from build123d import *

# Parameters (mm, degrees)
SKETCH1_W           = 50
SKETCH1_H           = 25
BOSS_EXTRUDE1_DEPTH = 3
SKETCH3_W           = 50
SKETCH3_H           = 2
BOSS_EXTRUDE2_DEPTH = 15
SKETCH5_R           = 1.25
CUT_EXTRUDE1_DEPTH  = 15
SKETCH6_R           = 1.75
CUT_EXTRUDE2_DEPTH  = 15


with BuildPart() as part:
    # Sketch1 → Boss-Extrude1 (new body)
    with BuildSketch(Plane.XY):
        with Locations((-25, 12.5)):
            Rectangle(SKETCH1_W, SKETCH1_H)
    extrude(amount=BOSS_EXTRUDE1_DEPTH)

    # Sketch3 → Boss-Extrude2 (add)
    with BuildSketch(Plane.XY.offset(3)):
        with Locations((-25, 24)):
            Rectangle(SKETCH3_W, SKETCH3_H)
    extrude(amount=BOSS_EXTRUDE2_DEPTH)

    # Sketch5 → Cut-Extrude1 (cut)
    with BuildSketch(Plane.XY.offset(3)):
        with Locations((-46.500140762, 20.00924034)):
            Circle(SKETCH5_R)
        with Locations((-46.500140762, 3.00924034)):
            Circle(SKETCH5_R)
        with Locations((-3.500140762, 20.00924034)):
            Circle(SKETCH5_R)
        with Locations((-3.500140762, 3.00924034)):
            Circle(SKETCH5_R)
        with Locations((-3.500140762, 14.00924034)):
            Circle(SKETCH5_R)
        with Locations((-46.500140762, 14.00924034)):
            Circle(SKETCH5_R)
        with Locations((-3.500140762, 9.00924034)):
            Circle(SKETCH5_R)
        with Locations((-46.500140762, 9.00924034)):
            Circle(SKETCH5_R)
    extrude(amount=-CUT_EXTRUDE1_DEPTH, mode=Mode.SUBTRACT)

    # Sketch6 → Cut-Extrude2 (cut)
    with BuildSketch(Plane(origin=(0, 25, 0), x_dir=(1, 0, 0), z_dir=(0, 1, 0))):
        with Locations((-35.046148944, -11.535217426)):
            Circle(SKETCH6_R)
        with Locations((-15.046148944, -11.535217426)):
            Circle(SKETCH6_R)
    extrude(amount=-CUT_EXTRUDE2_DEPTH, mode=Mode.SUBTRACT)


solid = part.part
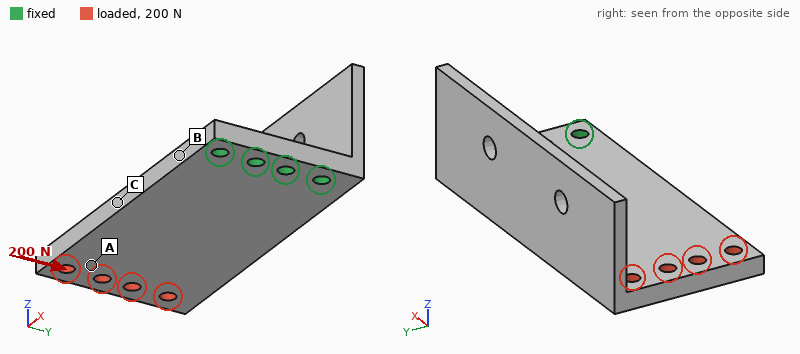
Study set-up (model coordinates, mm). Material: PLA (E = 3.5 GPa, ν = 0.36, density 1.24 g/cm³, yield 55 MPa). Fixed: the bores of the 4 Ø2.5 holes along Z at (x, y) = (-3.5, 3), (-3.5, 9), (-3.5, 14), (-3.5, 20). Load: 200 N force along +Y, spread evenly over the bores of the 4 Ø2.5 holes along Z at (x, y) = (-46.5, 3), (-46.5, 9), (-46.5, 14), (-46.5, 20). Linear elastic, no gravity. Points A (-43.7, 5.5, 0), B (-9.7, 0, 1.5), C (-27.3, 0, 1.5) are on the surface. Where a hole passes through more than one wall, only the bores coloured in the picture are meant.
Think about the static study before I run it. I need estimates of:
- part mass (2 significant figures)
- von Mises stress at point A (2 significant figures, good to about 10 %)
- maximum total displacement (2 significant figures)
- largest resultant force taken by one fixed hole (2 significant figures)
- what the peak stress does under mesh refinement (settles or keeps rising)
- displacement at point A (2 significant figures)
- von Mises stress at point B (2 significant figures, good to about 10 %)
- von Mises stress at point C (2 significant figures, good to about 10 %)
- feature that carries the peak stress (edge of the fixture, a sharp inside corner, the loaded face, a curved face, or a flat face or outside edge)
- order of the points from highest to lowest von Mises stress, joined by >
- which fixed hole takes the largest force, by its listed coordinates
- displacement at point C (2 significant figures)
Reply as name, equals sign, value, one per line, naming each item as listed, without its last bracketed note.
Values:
part mass = 6.3 g
von Mises stress at point A = 4.5 MPa
maximum total displacement = 0.60 mm
largest resultant force taken by one fixed hole = 470 N
what the peak stress does under mesh refinement = keeps rising
displacement at point A = 0.48 mm
von Mises stress at point B = 22 MPa
von Mises stress at point C = 11 MPa
feature that carries the peak stress = edge of the fixture
order of the points from highest to lowest von Mises stress, joined by > = B > C > A
which fixed hole takes the largest force, by its listed coordinates = (-3.5, 20)
displacement at point C = 0.26 mm
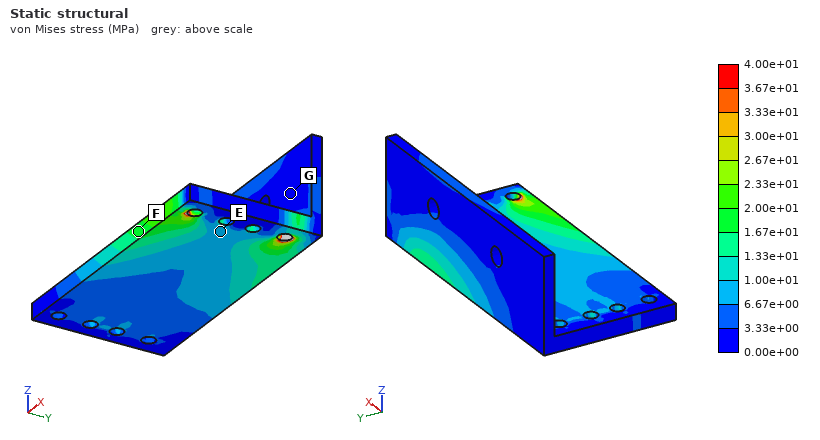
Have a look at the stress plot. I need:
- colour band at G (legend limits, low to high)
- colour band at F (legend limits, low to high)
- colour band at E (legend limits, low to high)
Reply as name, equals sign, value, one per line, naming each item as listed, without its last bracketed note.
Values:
colour band at G = 0.00e+00 to 3.33e+00 MPa
colour band at F = 1.67e+01 to 2.00e+01 MPa
colour band at E = 6.67e+00 to 1.00e+01 MPa
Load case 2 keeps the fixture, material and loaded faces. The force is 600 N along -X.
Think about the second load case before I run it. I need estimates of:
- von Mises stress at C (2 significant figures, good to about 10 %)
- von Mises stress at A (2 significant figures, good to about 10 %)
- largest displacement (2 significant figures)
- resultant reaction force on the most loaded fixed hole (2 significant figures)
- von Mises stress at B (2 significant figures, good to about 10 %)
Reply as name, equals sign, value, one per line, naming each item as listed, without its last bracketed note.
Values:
von Mises stress at C = 10 MPa
von Mises stress at A = 9.2 MPa
largest displacement = 0.15 mm
resultant reaction force on the most loaded fixed hole = 180 N
von Mises stress at B = 8.6 MPa
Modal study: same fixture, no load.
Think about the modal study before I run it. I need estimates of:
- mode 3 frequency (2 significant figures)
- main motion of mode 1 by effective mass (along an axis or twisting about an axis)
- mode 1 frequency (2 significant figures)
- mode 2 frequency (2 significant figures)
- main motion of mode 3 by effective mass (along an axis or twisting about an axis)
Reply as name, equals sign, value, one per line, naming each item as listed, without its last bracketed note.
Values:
mode 3 frequency = 2000 Hz
main motion of mode 1 by effective mass = along Z
mode 1 frequency = 520 Hz
mode 2 frequency = 990 Hz
main motion of mode 3 by effective mass = along Y
